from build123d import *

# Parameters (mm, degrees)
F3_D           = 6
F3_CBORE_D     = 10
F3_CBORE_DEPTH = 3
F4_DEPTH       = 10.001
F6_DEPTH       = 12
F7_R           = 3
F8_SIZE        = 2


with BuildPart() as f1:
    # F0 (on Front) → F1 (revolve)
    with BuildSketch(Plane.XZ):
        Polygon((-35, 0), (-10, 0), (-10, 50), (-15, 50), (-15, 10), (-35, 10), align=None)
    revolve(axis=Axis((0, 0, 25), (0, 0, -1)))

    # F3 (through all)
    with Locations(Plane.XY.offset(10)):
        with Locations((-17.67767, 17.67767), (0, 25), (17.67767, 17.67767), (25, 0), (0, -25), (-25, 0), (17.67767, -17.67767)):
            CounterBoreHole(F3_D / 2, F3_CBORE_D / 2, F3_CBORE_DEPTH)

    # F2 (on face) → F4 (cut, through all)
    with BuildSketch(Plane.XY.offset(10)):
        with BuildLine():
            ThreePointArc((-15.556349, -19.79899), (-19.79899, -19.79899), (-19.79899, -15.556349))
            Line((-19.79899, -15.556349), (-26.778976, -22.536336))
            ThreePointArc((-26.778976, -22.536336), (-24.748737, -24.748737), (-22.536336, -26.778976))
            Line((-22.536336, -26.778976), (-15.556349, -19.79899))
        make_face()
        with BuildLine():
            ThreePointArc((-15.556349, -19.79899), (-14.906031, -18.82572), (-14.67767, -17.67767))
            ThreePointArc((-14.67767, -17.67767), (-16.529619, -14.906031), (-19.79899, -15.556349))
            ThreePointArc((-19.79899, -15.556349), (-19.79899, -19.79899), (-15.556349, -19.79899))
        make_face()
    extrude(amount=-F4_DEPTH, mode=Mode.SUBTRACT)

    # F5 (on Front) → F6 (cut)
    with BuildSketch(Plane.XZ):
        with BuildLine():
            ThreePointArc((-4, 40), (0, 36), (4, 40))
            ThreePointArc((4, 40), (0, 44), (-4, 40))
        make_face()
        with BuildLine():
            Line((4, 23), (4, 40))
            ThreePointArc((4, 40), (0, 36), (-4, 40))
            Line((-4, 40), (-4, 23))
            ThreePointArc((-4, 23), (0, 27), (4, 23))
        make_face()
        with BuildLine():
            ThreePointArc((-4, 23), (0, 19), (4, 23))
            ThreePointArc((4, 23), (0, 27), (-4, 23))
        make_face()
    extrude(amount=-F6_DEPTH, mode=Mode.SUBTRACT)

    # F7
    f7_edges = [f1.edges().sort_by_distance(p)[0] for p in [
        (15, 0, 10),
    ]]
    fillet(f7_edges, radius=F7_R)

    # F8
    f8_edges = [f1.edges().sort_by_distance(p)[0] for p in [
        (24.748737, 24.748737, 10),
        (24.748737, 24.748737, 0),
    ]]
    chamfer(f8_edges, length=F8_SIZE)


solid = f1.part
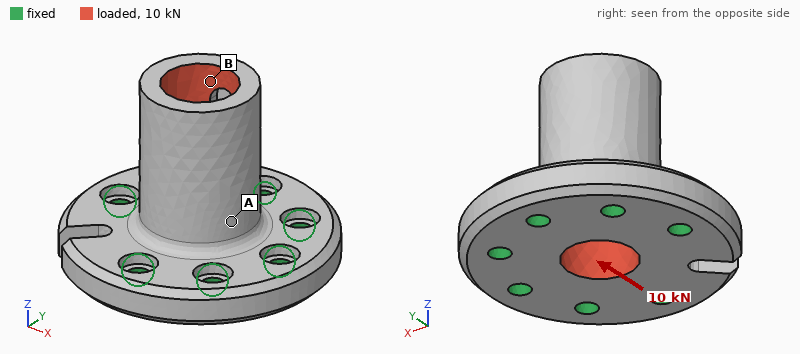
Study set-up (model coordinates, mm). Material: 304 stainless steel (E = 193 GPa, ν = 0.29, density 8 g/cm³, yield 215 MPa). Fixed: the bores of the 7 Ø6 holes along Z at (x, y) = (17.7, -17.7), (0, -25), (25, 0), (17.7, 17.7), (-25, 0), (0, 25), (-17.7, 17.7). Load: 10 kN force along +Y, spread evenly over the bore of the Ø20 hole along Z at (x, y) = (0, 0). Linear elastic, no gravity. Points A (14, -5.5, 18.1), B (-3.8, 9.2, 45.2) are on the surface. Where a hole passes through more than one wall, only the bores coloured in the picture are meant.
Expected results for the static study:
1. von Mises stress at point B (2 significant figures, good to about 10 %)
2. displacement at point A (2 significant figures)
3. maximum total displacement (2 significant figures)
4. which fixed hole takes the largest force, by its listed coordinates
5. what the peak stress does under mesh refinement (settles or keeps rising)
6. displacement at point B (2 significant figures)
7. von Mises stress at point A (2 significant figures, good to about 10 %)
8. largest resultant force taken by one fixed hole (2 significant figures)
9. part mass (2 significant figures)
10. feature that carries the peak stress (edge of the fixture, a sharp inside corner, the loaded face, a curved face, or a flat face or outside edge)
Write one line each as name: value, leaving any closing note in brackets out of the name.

von Mises stress at point B: 15 MPa
displacement at point A: 7.1 µm
maximum total displacement: 34 µm
which fixed hole takes the largest force, by its listed coordinates: (0, -25)
what the peak stress does under mesh refinement: keeps rising
displacement at point B: 28 µm
von Mises stress at point A: 35 MPa
largest resultant force taken by one fixed hole: 4.5 kN
part mass: 370 g
feature that carries the peak stress: edge of the fixture
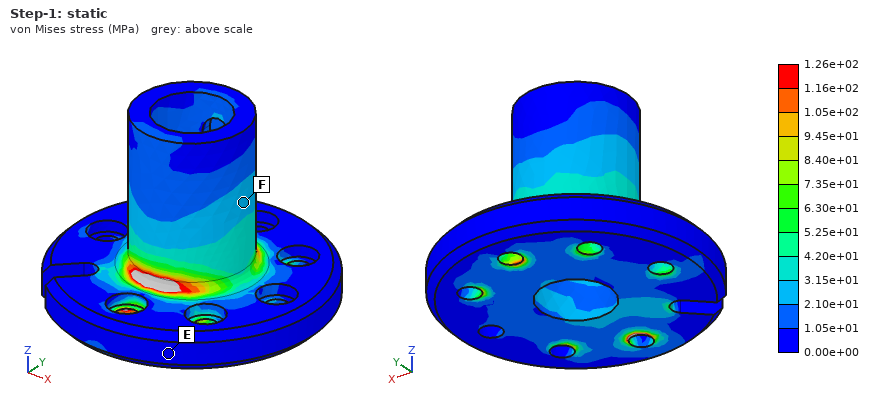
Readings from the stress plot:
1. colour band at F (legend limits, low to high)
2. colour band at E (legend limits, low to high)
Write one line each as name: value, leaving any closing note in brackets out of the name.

colour band at F: 2.10e+01 to 3.15e+01 MPa
colour band at E: 0.00e+00 to 1.05e+01 MPa
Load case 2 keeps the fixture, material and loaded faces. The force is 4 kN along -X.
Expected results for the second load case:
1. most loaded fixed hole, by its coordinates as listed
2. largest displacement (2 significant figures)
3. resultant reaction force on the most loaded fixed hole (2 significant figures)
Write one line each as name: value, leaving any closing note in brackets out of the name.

most loaded fixed hole, by its coordinates as listed: (-25, 0)
largest displacement: 14 µm
resultant reaction force on the most loaded fixed hole: 1.8 kN
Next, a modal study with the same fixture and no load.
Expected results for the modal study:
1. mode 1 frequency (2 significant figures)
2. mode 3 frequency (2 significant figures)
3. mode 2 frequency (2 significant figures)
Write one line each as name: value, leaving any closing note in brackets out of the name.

mode 1 frequency: 8000 Hz
mode 3 frequency: 18 kHz
mode 2 frequency: 8400 Hz
